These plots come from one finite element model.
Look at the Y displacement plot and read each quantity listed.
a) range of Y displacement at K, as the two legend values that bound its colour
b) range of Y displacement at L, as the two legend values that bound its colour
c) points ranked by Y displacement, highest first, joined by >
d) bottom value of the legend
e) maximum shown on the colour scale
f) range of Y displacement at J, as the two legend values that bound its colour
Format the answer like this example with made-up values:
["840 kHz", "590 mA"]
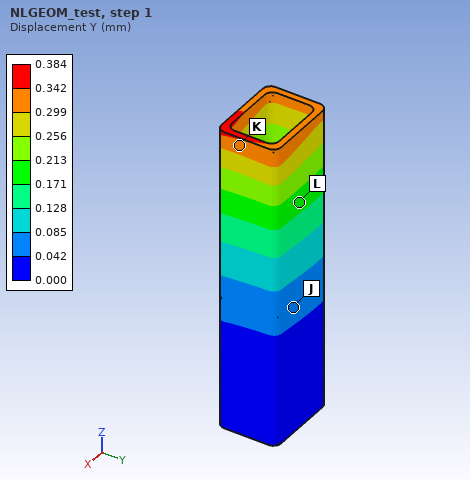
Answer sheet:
["0.299 to 0.342 mm", "0.171 to 0.213 mm", "K > L > J", "0.000 mm", "0.384 mm", "0.042 to 0.085 mm"]
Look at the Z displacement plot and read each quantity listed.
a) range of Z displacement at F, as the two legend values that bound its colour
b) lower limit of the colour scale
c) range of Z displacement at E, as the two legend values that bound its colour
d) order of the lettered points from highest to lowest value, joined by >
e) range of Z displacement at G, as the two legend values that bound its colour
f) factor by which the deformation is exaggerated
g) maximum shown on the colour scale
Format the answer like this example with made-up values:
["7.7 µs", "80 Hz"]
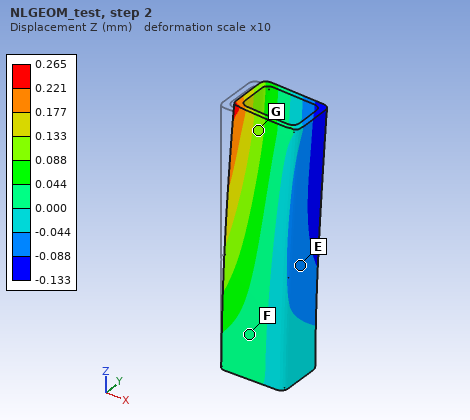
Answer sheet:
["0.000 to 0.044 mm", "-0.133 mm", "-0.088 to -0.044 mm", "G > F > E", "0.088 to 0.133 mm", "10", "0.265 mm"]
